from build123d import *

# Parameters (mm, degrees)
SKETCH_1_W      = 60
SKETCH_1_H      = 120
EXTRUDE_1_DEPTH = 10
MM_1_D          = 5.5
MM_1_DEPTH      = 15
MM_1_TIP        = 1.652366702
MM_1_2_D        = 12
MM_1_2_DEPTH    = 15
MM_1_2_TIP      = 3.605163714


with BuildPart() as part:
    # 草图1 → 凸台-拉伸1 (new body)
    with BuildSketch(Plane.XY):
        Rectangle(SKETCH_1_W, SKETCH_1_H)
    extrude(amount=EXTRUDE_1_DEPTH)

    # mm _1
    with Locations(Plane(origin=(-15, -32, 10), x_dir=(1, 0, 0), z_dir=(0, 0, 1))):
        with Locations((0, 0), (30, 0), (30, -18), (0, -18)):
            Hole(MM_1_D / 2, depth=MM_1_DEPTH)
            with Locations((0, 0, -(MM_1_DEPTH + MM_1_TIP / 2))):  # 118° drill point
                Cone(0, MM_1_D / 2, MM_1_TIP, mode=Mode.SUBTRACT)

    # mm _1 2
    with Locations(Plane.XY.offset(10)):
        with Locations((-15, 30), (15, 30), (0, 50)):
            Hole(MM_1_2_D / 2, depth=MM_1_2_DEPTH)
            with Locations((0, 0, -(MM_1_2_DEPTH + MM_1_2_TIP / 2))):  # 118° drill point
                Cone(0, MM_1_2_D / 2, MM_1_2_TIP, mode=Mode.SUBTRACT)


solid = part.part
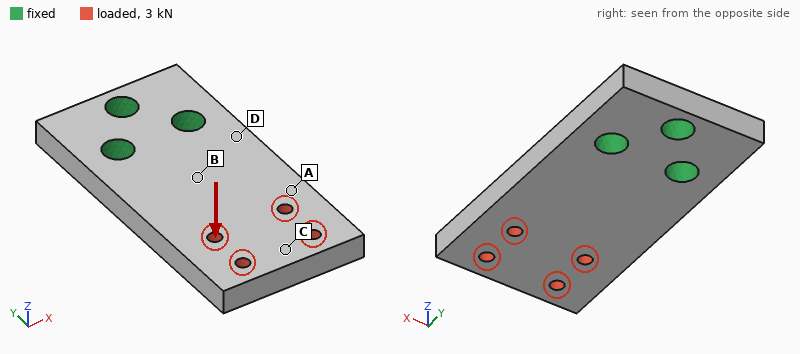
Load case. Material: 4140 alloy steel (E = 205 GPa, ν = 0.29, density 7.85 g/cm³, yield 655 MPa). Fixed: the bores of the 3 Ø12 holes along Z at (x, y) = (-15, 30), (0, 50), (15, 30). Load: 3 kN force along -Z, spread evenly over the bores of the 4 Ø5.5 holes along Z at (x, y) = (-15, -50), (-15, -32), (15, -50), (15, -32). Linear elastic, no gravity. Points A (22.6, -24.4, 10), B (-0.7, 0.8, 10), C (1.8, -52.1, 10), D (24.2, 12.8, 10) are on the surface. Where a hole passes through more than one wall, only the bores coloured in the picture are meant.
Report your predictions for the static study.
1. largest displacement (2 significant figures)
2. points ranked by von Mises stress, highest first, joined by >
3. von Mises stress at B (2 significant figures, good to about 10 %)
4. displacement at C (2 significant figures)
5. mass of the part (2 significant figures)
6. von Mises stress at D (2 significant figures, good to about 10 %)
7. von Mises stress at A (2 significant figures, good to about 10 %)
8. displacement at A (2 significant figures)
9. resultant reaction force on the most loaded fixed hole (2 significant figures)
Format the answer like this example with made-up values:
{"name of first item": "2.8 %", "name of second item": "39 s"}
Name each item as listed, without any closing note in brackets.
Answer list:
{"largest displacement": "0.43 mm", "points ranked by von Mises stress, highest first, joined by >": "D > B > A > C", "von Mises stress at B": "120 MPa", "displacement at C": "0.38 mm", "mass of the part": "530 g", "von Mises stress at D": "150 MPa", "von Mises stress at A": "54 MPa", "displacement at A": "0.19 mm", "resultant reaction force on the most loaded fixed hole": "1.9 kN"}
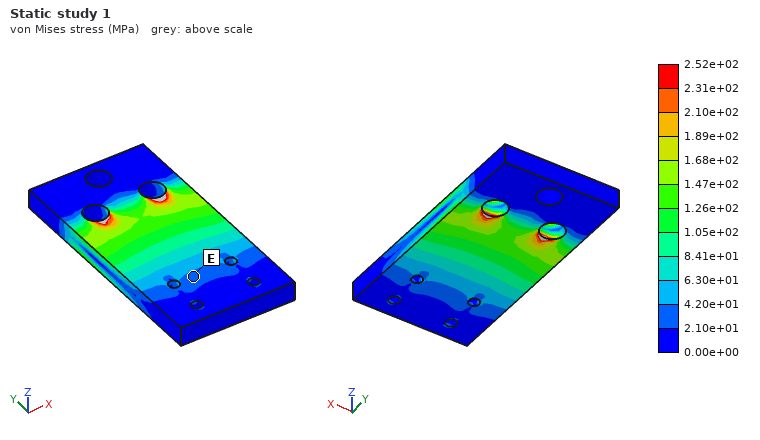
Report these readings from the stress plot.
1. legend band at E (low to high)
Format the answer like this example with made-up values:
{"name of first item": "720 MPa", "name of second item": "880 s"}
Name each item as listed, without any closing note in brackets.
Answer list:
{"legend band at E": "2.10e+01 to 4.20e+01 MPa"}
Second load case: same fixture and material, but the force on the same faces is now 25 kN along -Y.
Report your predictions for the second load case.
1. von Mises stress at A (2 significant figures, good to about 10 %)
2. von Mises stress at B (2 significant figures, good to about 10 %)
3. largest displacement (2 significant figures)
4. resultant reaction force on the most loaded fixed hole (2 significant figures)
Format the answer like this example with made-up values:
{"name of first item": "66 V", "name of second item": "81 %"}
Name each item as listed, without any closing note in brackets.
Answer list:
{"von Mises stress at A": "43 MPa", "von Mises stress at B": "43 MPa", "largest displacement": "16 µm", "resultant reaction force on the most loaded fixed hole": "12 kN"}
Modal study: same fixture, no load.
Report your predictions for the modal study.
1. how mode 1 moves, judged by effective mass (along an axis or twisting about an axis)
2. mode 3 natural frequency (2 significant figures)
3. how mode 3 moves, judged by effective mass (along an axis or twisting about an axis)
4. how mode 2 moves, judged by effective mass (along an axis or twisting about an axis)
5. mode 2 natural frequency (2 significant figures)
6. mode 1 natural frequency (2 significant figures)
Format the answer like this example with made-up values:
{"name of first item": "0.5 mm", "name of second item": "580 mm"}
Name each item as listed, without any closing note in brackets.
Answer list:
{"how mode 1 moves, judged by effective mass": "along Z", "mode 3 natural frequency": "4800 Hz", "how mode 3 moves, judged by effective mass": "along X", "how mode 2 moves, judged by effective mass": "twisting about Y", "mode 2 natural frequency": "3400 Hz", "mode 1 natural frequency": "1100 Hz"}
